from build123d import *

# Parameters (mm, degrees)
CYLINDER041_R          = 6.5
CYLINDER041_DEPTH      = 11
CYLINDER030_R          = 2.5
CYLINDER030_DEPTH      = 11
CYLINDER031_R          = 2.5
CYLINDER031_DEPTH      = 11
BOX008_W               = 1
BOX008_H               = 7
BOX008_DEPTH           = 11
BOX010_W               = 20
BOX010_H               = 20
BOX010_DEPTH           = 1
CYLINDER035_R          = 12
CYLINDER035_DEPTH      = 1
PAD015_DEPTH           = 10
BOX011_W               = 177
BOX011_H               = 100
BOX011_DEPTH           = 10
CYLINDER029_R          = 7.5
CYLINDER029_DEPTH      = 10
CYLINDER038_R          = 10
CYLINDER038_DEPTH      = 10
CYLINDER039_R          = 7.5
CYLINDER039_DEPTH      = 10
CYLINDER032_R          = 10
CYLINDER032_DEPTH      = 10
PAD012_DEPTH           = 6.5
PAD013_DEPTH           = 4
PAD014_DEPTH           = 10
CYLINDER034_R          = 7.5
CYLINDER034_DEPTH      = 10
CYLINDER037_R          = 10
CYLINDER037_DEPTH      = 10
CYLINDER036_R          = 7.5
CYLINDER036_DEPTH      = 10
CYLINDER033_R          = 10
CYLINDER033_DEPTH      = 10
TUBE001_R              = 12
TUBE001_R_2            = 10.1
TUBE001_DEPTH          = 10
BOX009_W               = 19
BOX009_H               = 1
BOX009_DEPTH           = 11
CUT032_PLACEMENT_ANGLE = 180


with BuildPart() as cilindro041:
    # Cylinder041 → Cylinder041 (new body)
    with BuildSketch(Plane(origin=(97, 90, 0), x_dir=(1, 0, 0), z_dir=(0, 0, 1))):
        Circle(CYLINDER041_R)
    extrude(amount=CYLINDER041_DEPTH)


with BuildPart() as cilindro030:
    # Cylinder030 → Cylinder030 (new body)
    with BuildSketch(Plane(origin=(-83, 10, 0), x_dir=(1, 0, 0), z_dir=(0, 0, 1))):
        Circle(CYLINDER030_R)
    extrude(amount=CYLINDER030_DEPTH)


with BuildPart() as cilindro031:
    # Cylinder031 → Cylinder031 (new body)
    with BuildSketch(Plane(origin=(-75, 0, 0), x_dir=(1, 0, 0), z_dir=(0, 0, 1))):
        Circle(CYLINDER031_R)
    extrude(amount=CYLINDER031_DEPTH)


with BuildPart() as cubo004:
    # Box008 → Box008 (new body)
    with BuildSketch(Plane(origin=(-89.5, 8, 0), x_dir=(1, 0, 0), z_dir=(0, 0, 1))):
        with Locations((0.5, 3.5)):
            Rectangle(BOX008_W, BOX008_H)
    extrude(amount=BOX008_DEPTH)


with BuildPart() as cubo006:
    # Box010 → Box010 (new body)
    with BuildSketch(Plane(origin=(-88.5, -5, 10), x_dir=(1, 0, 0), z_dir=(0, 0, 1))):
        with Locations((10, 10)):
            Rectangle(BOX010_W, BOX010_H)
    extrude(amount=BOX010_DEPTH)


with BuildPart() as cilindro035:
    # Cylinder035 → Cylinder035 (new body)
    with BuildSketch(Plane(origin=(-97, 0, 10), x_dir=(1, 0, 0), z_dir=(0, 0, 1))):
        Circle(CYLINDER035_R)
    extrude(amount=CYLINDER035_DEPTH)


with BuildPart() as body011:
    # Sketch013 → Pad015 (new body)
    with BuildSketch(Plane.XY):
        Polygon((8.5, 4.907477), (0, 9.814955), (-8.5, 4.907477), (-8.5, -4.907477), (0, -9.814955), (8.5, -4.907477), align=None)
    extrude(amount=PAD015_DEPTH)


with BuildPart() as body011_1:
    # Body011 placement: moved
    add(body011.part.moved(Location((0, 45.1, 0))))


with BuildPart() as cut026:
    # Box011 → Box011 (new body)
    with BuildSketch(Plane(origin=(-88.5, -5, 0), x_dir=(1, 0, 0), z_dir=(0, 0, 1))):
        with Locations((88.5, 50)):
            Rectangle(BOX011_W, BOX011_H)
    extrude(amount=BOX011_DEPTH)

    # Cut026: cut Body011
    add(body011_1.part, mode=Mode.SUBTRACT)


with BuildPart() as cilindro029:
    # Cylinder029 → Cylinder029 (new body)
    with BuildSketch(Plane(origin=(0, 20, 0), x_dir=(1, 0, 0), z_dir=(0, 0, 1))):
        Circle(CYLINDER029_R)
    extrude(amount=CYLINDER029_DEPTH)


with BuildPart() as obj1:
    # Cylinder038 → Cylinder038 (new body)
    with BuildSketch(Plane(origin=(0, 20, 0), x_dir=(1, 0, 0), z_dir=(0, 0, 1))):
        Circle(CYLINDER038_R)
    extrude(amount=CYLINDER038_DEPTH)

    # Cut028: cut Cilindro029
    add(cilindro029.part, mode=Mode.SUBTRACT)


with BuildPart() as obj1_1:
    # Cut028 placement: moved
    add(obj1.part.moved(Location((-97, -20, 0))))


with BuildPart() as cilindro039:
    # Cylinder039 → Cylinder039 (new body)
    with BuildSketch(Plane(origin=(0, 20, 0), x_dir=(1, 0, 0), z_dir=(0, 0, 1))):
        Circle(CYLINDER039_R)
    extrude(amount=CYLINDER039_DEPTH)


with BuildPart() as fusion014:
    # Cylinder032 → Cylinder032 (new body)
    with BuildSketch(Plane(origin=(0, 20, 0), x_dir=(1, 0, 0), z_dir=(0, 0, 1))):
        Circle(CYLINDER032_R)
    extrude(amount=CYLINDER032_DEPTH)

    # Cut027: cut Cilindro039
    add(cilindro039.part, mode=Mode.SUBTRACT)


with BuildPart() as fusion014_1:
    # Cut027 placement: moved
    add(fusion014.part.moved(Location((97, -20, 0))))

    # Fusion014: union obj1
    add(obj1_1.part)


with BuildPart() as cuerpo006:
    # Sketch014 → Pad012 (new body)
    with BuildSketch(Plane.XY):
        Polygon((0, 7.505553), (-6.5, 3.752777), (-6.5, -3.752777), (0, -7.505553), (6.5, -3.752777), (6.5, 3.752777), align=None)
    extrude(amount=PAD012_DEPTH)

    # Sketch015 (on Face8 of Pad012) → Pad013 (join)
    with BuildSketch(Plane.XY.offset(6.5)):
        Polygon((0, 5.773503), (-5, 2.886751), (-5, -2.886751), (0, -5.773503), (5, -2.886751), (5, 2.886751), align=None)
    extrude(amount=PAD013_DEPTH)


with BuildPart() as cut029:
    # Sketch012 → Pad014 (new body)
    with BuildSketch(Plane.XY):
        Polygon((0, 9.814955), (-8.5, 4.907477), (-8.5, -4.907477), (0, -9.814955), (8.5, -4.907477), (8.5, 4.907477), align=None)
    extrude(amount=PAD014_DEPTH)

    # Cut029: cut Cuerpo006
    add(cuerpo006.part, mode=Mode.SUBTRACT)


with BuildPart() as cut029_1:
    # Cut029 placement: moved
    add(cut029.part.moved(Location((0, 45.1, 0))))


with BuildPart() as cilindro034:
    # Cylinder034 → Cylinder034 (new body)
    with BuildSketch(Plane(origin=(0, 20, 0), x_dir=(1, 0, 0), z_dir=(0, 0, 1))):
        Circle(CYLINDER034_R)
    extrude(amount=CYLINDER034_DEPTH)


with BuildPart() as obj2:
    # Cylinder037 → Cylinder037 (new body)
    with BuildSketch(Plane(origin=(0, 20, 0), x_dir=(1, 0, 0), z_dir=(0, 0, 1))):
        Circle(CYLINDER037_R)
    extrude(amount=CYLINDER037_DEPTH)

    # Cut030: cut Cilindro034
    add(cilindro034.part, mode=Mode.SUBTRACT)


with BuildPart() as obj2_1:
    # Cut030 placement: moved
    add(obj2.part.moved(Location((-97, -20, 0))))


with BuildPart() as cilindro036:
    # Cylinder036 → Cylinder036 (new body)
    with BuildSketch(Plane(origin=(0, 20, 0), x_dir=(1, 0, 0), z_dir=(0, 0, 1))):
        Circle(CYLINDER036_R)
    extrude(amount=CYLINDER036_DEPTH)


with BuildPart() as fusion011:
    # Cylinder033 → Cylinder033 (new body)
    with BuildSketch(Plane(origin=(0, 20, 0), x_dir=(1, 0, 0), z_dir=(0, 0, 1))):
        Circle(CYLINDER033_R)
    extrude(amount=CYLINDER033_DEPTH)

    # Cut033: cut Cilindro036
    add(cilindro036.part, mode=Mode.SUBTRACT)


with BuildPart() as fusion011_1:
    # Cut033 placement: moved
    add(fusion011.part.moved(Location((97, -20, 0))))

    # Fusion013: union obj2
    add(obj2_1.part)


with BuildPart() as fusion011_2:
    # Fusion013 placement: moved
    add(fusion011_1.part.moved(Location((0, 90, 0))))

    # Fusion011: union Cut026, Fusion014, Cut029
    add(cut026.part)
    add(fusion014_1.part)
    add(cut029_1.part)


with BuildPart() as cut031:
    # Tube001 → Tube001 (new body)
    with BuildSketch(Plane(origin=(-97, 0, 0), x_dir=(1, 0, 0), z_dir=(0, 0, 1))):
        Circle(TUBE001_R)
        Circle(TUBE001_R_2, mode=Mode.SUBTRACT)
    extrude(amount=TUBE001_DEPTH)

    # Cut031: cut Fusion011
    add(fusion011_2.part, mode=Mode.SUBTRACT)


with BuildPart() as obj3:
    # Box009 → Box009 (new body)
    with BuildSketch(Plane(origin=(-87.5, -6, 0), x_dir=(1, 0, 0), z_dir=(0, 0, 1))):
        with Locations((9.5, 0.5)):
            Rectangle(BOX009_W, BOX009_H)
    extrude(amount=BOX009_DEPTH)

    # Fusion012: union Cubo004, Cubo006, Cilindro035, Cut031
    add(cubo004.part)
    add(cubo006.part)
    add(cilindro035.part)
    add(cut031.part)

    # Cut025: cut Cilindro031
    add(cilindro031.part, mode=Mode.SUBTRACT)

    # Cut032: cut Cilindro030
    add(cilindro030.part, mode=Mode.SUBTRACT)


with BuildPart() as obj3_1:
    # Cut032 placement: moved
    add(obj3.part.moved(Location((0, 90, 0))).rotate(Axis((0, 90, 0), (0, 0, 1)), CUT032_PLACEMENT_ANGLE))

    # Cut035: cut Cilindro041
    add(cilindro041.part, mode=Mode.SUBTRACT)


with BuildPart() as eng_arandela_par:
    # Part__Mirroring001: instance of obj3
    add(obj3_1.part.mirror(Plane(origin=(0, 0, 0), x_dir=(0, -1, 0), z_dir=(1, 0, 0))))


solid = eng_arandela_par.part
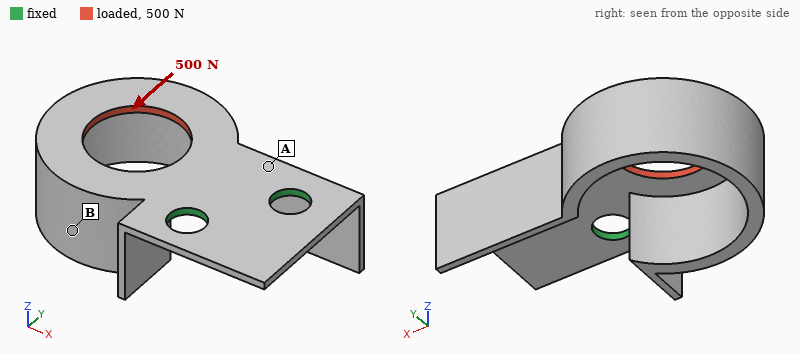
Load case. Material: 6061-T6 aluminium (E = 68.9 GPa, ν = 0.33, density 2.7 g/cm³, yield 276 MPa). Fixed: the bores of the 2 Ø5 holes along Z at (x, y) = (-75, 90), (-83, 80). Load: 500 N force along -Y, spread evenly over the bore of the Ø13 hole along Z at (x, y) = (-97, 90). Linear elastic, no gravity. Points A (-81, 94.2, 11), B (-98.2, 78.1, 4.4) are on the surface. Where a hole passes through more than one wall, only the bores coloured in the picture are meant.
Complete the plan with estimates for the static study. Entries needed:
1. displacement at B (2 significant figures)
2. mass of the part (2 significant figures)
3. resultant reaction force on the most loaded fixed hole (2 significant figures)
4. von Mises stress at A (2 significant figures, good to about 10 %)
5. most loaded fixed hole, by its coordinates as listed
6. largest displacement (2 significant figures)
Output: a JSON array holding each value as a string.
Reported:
["0.071 mm", "5.4 g", "720 N", "56 MPa", "(-83, 80)", "0.12 mm"]
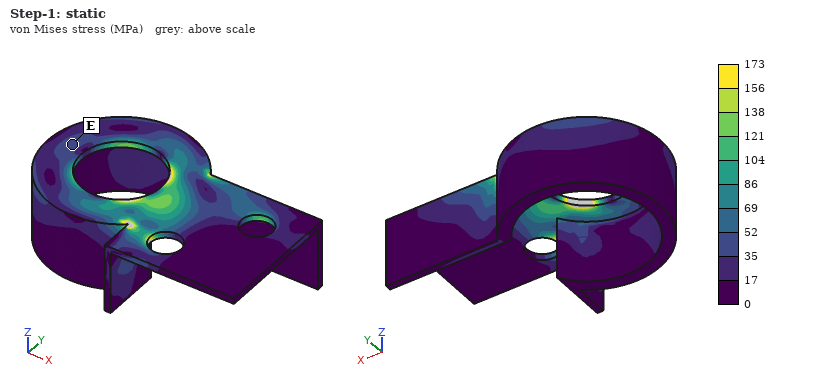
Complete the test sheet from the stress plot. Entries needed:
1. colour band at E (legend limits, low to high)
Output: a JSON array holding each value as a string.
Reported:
["35 to 52 MPa"]
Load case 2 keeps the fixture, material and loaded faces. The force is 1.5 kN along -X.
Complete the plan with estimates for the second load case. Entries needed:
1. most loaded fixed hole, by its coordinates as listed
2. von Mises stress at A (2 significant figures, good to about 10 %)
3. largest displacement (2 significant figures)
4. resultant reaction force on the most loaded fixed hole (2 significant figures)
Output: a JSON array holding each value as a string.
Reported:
["(-75, 90)", "130 MPa", "0.13 mm", "1.1 kN"]
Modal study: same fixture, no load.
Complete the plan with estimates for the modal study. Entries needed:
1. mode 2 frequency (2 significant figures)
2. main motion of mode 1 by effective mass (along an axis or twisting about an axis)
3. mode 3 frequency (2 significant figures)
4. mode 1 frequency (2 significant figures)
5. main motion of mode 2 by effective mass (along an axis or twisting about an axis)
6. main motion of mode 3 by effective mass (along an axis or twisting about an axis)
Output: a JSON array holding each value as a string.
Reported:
["2700 Hz", "along Z", "5700 Hz", "1100 Hz", "along Y", "along Y"]
